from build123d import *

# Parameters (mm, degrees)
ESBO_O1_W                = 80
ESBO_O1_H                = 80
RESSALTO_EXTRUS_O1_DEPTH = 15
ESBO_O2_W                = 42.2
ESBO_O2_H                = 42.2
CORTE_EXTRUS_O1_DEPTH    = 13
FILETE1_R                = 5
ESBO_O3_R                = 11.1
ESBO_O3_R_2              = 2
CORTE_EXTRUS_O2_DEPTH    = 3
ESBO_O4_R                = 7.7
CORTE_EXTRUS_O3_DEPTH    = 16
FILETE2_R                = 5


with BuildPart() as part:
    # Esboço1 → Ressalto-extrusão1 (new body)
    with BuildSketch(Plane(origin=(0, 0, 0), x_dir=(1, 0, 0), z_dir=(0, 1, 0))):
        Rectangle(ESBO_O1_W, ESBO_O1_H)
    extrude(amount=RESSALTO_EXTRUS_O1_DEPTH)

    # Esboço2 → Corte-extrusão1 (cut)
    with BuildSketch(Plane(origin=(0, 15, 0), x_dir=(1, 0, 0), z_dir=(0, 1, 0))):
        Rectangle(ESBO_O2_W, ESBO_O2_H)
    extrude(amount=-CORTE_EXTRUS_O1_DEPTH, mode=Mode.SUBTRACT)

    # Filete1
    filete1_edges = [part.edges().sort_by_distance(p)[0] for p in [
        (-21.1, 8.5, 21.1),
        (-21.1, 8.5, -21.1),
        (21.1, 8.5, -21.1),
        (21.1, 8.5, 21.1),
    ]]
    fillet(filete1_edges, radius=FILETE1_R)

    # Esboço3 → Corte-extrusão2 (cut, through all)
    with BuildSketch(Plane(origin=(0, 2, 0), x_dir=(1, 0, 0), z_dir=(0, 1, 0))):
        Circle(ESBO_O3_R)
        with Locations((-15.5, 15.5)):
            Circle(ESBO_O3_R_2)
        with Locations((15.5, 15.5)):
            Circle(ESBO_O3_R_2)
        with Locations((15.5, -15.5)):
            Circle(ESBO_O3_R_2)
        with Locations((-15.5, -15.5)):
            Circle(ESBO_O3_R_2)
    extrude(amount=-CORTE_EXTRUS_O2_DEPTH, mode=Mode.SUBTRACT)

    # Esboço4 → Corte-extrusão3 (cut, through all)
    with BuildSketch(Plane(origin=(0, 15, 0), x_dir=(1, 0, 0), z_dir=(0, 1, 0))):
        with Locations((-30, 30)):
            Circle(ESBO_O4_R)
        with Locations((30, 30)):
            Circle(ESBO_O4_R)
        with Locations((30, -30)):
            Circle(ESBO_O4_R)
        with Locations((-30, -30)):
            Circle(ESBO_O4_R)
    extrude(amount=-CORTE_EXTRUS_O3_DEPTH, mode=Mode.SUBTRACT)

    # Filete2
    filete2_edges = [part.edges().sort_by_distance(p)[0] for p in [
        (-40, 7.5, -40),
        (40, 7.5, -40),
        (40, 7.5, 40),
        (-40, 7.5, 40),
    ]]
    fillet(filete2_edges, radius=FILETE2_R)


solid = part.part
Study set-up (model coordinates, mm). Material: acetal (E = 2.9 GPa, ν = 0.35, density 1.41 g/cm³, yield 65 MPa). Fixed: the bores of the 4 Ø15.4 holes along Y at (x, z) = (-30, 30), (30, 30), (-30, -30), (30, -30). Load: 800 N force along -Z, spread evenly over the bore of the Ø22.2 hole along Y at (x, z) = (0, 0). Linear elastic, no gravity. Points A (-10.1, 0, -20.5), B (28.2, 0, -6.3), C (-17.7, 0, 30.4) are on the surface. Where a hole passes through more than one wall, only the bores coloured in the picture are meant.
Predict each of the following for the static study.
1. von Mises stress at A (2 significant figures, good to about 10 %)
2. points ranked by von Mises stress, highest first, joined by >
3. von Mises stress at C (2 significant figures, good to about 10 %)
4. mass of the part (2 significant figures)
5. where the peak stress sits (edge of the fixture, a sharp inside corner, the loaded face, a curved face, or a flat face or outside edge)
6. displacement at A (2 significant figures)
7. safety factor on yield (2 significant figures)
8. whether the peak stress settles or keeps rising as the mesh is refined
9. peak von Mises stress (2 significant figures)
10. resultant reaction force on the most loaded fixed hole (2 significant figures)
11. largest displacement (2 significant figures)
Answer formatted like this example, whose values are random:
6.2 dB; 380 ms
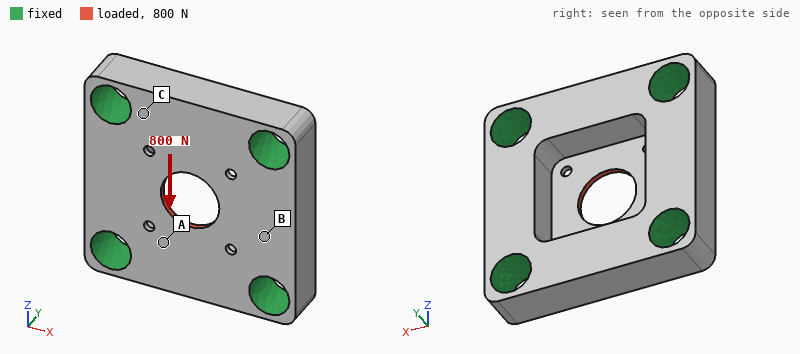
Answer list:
3.6 MPa; A > C > B; 2.1 MPa; 86 g; the loaded face; 23 µm; 6.1; settles; 11 MPa; 220 N; 50 µm
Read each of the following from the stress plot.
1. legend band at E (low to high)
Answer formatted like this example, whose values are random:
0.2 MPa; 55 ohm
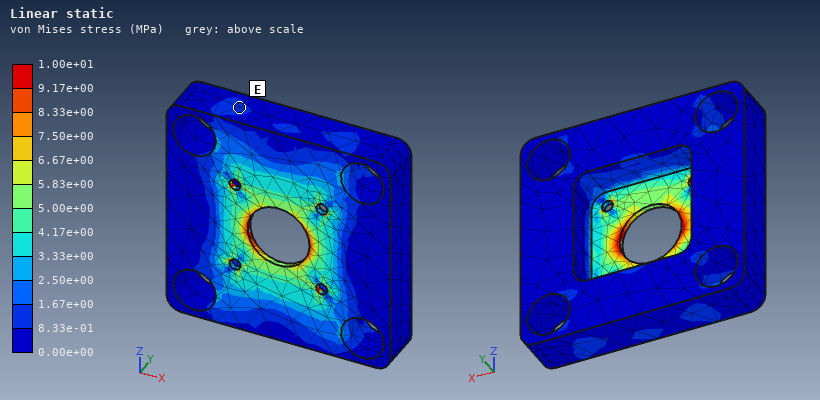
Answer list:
8.33e-01 to 1.67e+00 MPa
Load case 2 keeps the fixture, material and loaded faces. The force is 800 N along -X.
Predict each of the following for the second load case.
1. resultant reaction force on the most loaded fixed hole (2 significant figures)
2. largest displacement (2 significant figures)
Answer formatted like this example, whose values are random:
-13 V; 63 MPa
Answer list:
220 N; 50 µm
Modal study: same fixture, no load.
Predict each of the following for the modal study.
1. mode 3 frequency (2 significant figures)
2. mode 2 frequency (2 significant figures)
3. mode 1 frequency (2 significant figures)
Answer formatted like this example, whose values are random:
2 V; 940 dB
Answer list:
4700 Hz; 4700 Hz; 3800 Hz
